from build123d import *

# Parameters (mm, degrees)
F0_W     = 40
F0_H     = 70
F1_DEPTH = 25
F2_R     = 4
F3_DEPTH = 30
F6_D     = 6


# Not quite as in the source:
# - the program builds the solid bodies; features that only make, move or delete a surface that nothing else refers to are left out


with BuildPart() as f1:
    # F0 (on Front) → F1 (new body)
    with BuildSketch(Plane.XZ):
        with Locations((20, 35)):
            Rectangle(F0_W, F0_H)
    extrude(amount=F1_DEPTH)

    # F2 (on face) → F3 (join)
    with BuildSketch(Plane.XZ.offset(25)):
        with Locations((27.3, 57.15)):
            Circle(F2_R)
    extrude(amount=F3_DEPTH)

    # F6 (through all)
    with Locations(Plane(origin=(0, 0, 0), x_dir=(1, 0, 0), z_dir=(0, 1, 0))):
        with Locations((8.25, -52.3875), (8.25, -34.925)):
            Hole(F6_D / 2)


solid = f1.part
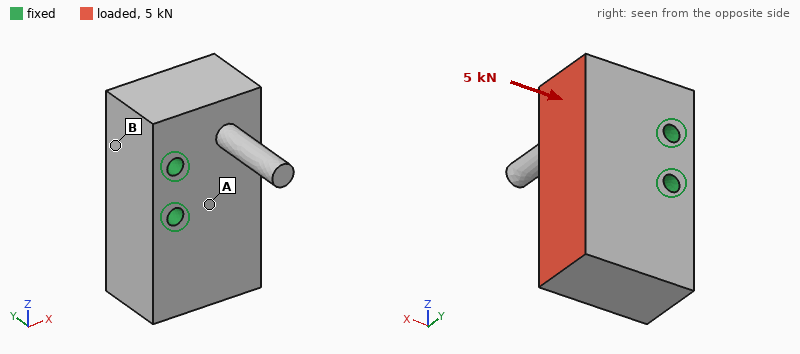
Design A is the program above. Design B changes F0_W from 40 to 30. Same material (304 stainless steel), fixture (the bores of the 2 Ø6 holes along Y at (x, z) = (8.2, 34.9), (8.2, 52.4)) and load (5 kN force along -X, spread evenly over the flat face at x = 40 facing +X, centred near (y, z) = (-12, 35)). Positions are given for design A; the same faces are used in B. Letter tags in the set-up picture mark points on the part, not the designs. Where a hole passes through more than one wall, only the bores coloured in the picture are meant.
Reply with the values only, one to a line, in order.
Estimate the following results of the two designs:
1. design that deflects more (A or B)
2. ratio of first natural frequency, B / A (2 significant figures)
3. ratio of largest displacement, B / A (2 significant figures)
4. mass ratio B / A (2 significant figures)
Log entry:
B
0.99
1.3
0.75
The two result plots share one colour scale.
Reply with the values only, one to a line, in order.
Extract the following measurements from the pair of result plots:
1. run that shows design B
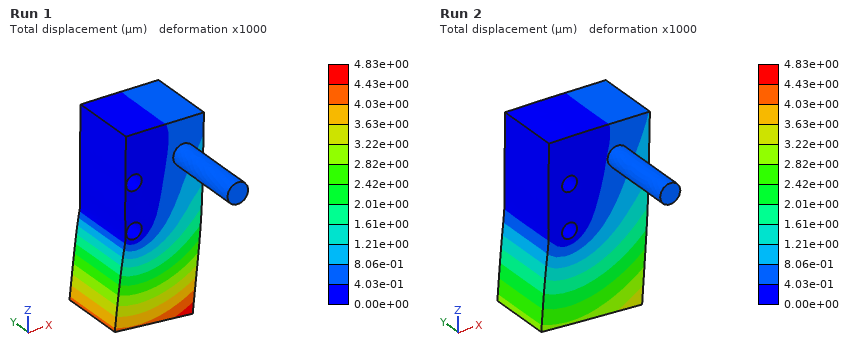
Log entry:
Run 1
